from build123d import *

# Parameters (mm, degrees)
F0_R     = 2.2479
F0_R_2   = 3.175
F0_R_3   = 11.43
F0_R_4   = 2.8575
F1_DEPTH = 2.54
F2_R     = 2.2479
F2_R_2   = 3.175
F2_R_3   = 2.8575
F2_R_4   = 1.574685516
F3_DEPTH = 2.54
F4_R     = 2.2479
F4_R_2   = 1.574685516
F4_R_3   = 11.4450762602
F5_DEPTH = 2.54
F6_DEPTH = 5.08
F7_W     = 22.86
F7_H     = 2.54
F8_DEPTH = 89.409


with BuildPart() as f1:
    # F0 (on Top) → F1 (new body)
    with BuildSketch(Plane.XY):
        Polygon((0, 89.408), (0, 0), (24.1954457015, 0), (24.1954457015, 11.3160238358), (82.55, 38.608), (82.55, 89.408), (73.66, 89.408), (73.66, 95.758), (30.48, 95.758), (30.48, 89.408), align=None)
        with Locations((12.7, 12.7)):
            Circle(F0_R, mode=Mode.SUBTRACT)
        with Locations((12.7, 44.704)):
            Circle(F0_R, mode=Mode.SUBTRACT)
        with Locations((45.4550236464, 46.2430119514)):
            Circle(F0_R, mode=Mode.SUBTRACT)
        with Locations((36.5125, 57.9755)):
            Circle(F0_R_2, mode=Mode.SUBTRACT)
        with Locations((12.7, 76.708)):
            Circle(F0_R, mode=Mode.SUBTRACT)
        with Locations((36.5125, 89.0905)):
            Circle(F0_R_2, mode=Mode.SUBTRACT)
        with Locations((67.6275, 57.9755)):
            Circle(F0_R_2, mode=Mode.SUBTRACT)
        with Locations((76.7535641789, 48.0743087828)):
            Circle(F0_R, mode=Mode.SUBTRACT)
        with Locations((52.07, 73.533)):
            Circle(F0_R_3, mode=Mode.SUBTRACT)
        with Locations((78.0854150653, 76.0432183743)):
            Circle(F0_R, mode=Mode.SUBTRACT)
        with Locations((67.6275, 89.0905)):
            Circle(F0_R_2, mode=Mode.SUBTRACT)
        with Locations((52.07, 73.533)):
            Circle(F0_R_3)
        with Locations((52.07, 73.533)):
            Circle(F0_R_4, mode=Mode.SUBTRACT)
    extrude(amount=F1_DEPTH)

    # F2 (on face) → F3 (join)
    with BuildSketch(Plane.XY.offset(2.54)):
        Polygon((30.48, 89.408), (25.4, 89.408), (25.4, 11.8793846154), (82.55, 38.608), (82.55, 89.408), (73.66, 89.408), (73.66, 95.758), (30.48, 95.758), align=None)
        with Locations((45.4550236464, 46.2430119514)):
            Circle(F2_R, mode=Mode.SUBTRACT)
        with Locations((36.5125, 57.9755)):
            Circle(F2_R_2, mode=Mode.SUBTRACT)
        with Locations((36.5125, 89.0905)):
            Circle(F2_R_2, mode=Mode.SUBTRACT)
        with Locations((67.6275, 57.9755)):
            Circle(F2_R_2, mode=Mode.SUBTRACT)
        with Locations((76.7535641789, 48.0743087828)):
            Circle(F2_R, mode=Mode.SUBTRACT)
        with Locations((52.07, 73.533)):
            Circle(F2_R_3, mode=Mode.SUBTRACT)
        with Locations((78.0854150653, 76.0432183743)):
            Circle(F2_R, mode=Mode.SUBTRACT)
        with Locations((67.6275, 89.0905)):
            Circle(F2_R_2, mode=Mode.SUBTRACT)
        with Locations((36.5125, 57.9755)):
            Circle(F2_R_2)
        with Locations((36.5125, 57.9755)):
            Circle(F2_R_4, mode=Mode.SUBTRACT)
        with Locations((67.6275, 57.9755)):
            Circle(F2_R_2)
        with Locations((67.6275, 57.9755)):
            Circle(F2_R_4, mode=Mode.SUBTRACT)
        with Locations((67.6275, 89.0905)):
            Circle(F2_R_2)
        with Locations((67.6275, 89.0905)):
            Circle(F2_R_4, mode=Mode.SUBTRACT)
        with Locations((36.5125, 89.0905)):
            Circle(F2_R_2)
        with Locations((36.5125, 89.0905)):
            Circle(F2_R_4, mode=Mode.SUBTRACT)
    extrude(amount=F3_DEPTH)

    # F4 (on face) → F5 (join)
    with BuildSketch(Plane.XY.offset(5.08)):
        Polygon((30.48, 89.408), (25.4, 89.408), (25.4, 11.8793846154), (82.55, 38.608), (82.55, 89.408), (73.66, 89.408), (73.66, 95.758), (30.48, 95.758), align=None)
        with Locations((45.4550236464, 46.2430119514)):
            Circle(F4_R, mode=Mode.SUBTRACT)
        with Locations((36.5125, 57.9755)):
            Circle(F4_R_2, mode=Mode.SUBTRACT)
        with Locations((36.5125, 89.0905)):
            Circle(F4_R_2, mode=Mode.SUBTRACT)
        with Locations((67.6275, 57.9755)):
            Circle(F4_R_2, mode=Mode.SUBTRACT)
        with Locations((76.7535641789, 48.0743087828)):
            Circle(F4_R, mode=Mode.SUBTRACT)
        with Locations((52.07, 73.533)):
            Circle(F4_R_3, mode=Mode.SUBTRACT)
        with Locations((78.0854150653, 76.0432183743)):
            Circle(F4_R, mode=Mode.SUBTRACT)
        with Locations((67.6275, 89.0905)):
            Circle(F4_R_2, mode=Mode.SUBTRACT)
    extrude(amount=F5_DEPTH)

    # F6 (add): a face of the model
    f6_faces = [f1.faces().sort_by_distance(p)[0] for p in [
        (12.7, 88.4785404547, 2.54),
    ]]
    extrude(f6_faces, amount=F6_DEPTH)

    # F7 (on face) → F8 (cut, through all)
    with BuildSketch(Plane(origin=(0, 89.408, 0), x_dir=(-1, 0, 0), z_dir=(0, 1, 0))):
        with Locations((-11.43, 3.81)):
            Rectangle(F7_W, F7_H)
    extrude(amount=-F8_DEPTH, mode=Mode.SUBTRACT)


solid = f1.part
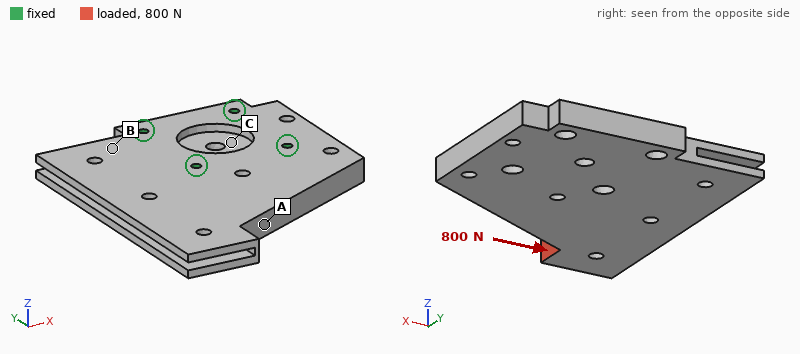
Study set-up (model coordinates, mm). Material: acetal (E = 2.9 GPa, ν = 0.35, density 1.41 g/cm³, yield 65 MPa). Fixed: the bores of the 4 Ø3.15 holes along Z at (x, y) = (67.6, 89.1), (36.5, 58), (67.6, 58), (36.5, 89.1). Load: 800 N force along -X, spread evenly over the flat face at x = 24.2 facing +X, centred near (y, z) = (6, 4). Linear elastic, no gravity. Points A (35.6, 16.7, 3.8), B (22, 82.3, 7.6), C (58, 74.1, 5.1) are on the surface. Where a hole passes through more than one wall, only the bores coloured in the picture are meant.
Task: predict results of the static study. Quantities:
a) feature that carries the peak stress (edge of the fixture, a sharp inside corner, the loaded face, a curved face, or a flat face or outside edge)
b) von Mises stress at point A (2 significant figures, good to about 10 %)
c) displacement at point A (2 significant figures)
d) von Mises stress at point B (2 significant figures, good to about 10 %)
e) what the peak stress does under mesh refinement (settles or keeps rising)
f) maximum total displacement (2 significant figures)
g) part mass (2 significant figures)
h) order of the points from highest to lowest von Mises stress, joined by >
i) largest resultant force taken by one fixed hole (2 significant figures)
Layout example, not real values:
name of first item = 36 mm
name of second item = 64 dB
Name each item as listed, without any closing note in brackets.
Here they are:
feature that carries the peak stress = edge of the fixture
von Mises stress at point A = 13 MPa
displacement at point A = 0.24 mm
von Mises stress at point B = 5.1 MPa
what the peak stress does under mesh refinement = keeps rising
maximum total displacement = 0.63 mm
part mass = 56 g
order of the points from highest to lowest von Mises stress, joined by > = A > B > C
largest resultant force taken by one fixed hole = 900 N
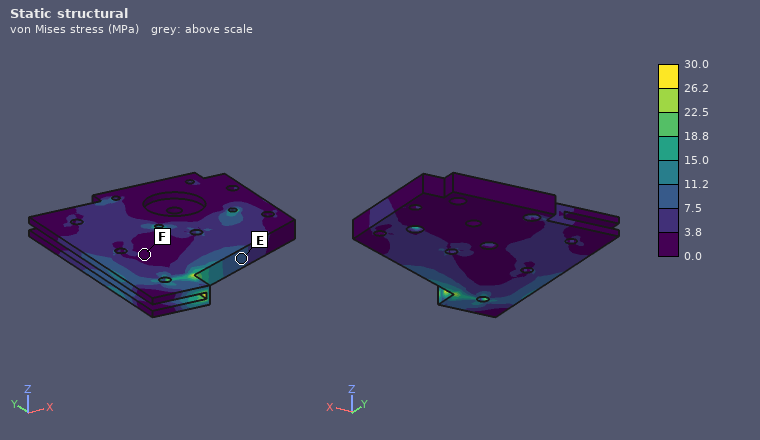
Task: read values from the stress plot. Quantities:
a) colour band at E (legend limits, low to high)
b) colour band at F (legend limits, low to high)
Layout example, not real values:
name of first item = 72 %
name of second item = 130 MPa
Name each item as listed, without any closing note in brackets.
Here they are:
colour band at E = 7.5 to 11.2 MPa
colour band at F = 0.0 to 3.8 MPa
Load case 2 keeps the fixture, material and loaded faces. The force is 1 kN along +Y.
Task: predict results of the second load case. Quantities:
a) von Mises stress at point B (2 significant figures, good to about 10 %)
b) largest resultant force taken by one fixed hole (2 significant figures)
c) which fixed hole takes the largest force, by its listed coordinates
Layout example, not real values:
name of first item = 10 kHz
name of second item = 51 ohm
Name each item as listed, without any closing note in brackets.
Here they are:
von Mises stress at point B = 3.1 MPa
largest resultant force taken by one fixed hole = 780 N
which fixed hole takes the largest force, by its listed coordinates = (36.5, 58)
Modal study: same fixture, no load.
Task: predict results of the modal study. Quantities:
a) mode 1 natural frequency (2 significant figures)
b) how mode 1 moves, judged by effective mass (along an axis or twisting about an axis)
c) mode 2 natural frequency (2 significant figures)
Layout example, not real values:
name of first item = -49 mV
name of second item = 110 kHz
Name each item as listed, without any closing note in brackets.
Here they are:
mode 1 natural frequency = 480 Hz
how mode 1 moves, judged by effective mass = along Z
mode 2 natural frequency = 880 Hz
